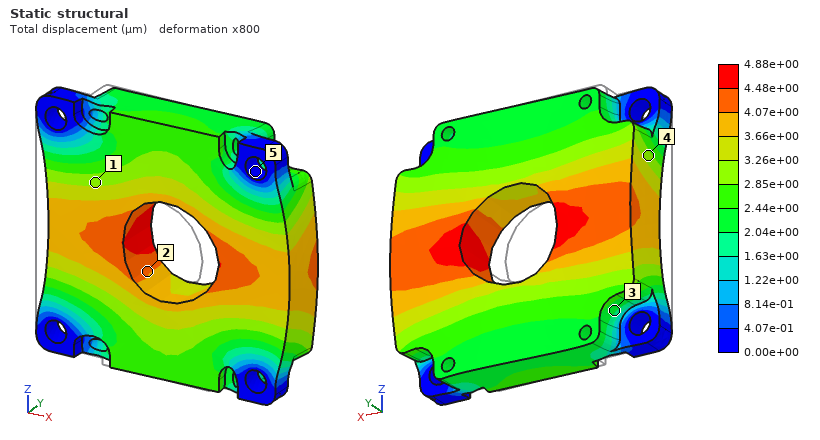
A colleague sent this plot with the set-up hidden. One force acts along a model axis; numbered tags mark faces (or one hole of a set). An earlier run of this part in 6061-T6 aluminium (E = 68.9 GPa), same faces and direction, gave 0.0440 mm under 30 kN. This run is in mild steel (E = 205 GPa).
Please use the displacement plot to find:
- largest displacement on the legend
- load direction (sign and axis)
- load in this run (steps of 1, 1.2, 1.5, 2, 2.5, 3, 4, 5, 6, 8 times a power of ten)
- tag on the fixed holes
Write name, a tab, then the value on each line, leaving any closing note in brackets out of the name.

largest displacement on the legend	4.88e+00 µm
load direction	+X
load in this run	10 kN
tag on the fixed holes	5
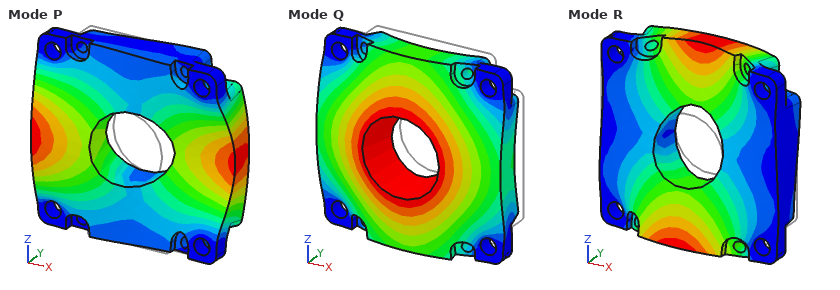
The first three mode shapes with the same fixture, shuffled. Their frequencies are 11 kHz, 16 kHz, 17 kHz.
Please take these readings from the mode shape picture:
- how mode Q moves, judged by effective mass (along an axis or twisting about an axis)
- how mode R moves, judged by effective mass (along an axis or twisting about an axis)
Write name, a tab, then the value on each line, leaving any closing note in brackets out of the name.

how mode Q moves, judged by effective mass	along Y
how mode R moves, judged by effective mass	twisting about X
